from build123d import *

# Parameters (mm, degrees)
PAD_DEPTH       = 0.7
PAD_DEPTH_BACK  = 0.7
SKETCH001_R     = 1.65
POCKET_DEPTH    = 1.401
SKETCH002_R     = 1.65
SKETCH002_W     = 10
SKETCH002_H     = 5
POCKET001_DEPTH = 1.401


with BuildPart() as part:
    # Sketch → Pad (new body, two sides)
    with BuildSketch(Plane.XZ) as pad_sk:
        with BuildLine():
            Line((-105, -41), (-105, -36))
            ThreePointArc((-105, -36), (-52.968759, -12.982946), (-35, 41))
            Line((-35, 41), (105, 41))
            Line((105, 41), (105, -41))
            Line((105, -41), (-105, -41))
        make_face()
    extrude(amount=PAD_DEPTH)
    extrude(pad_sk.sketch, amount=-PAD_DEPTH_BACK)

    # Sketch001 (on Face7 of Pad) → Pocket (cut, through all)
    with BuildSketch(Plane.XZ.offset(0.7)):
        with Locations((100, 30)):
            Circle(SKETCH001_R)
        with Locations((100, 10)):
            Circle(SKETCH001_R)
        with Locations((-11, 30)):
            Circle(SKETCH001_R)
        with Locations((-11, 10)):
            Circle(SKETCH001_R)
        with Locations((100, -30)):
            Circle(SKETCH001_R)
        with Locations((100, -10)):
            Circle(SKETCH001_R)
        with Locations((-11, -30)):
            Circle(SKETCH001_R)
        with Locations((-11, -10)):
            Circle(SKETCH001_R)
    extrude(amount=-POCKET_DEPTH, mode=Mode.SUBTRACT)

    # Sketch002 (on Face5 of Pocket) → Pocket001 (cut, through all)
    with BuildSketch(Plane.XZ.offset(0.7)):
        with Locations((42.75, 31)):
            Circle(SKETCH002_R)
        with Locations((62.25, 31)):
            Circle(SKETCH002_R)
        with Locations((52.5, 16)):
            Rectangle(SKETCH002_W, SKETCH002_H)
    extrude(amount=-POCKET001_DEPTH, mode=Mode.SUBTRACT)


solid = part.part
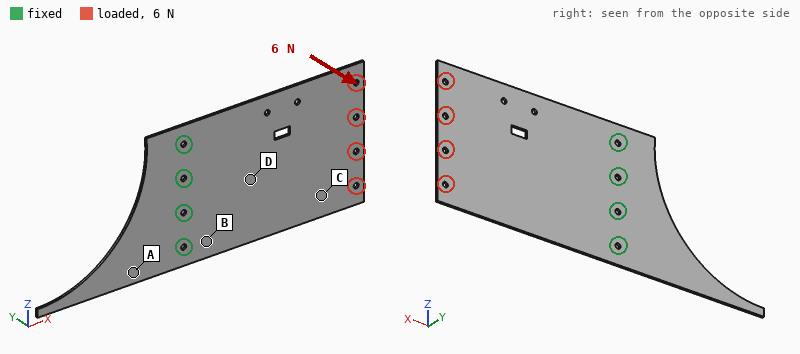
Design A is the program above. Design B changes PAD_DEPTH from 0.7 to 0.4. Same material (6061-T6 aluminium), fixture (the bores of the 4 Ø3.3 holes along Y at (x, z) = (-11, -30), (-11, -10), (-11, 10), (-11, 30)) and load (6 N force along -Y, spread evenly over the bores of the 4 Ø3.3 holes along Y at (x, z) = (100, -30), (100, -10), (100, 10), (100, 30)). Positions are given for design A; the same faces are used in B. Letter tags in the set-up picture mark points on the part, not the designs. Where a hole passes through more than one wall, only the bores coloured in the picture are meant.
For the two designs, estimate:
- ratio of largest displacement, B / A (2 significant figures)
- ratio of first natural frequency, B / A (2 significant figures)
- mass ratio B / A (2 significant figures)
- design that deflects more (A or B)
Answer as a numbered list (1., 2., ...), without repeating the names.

1. 2.1
2. 0.79
3. 0.79
4. B
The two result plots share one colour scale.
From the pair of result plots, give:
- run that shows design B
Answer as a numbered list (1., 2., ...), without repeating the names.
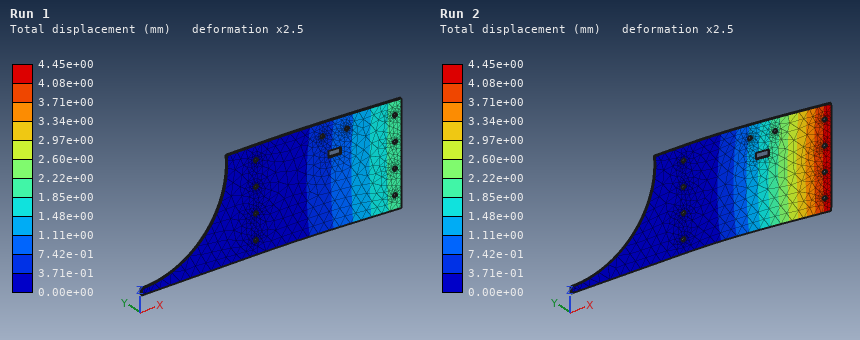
1. Run 2
